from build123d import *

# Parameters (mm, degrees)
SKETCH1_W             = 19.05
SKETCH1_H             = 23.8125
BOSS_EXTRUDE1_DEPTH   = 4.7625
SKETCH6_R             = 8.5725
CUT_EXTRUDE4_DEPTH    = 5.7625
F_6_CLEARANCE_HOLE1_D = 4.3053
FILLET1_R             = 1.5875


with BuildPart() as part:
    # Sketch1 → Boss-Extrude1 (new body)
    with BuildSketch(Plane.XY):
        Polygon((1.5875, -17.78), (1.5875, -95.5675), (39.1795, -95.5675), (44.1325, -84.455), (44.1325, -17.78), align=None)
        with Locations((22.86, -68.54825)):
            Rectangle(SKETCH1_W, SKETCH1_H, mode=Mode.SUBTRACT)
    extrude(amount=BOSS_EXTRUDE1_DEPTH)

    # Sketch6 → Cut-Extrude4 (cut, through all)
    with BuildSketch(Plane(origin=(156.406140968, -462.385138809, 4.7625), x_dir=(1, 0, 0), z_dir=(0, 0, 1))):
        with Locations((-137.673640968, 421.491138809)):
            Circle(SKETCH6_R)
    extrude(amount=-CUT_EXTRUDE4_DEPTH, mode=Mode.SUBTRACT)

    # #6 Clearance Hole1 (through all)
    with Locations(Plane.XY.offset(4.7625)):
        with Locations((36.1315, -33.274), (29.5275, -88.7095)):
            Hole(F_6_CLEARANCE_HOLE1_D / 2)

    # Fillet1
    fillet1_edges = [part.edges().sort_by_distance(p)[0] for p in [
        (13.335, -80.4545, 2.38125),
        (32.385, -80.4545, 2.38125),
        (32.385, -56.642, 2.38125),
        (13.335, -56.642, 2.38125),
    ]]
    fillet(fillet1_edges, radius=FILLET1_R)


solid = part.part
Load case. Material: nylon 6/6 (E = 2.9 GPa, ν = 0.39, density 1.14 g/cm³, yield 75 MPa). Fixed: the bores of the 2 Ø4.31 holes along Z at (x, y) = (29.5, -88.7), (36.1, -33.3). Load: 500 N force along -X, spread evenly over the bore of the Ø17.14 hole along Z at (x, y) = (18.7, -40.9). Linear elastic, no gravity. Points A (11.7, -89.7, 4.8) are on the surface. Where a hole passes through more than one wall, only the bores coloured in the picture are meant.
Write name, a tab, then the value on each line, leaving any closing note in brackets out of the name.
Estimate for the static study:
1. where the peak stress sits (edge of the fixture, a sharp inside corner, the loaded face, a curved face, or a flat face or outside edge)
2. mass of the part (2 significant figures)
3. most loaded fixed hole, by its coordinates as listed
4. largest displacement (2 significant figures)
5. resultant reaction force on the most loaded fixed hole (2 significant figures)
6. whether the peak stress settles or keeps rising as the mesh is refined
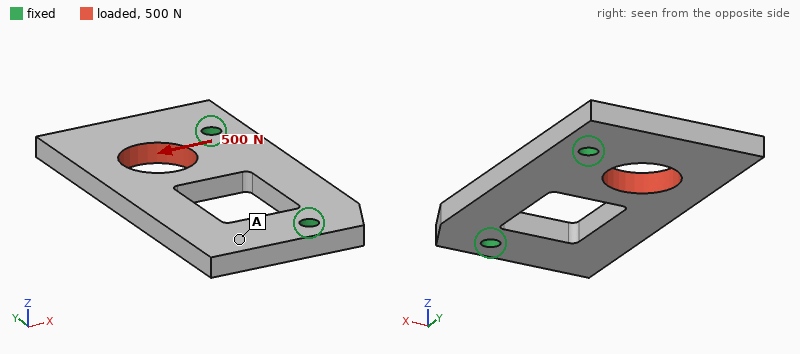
where the peak stress sits	edge of the fixture
mass of the part	14 g
most loaded fixed hole, by its coordinates as listed	(36.1, -33.3)
largest displacement	96 µm
resultant reaction force on the most loaded fixed hole	440 N
whether the peak stress settles or keeps rising as the mesh is refined	keeps rising
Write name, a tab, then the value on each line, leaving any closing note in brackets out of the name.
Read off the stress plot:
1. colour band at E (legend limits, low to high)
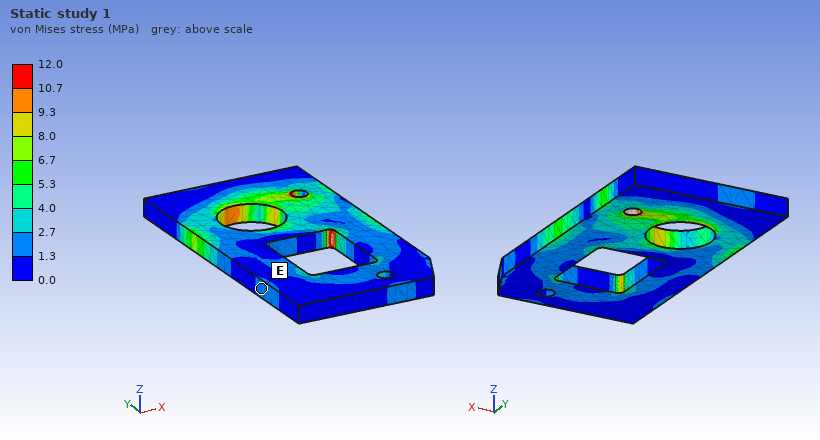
colour band at E	1.3 to 2.7 MPa
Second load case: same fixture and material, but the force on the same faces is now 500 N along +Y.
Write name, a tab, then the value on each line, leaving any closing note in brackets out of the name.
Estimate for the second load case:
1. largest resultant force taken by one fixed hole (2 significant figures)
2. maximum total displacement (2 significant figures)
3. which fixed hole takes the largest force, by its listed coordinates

largest resultant force taken by one fixed hole	350 N
maximum total displacement	0.18 mm
which fixed hole takes the largest force, by its listed coordinates	(36.1, -33.3)
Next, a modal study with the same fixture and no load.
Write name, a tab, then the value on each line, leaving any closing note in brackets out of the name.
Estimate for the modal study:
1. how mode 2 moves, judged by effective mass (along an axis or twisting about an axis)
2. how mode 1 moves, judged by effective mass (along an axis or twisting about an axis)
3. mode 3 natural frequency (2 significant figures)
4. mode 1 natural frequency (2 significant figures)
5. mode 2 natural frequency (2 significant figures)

how mode 2 moves, judged by effective mass	twisting about X
how mode 1 moves, judged by effective mass	along Z
mode 3 natural frequency	2100 Hz
mode 1 natural frequency	850 Hz
mode 2 natural frequency	1400 Hz
